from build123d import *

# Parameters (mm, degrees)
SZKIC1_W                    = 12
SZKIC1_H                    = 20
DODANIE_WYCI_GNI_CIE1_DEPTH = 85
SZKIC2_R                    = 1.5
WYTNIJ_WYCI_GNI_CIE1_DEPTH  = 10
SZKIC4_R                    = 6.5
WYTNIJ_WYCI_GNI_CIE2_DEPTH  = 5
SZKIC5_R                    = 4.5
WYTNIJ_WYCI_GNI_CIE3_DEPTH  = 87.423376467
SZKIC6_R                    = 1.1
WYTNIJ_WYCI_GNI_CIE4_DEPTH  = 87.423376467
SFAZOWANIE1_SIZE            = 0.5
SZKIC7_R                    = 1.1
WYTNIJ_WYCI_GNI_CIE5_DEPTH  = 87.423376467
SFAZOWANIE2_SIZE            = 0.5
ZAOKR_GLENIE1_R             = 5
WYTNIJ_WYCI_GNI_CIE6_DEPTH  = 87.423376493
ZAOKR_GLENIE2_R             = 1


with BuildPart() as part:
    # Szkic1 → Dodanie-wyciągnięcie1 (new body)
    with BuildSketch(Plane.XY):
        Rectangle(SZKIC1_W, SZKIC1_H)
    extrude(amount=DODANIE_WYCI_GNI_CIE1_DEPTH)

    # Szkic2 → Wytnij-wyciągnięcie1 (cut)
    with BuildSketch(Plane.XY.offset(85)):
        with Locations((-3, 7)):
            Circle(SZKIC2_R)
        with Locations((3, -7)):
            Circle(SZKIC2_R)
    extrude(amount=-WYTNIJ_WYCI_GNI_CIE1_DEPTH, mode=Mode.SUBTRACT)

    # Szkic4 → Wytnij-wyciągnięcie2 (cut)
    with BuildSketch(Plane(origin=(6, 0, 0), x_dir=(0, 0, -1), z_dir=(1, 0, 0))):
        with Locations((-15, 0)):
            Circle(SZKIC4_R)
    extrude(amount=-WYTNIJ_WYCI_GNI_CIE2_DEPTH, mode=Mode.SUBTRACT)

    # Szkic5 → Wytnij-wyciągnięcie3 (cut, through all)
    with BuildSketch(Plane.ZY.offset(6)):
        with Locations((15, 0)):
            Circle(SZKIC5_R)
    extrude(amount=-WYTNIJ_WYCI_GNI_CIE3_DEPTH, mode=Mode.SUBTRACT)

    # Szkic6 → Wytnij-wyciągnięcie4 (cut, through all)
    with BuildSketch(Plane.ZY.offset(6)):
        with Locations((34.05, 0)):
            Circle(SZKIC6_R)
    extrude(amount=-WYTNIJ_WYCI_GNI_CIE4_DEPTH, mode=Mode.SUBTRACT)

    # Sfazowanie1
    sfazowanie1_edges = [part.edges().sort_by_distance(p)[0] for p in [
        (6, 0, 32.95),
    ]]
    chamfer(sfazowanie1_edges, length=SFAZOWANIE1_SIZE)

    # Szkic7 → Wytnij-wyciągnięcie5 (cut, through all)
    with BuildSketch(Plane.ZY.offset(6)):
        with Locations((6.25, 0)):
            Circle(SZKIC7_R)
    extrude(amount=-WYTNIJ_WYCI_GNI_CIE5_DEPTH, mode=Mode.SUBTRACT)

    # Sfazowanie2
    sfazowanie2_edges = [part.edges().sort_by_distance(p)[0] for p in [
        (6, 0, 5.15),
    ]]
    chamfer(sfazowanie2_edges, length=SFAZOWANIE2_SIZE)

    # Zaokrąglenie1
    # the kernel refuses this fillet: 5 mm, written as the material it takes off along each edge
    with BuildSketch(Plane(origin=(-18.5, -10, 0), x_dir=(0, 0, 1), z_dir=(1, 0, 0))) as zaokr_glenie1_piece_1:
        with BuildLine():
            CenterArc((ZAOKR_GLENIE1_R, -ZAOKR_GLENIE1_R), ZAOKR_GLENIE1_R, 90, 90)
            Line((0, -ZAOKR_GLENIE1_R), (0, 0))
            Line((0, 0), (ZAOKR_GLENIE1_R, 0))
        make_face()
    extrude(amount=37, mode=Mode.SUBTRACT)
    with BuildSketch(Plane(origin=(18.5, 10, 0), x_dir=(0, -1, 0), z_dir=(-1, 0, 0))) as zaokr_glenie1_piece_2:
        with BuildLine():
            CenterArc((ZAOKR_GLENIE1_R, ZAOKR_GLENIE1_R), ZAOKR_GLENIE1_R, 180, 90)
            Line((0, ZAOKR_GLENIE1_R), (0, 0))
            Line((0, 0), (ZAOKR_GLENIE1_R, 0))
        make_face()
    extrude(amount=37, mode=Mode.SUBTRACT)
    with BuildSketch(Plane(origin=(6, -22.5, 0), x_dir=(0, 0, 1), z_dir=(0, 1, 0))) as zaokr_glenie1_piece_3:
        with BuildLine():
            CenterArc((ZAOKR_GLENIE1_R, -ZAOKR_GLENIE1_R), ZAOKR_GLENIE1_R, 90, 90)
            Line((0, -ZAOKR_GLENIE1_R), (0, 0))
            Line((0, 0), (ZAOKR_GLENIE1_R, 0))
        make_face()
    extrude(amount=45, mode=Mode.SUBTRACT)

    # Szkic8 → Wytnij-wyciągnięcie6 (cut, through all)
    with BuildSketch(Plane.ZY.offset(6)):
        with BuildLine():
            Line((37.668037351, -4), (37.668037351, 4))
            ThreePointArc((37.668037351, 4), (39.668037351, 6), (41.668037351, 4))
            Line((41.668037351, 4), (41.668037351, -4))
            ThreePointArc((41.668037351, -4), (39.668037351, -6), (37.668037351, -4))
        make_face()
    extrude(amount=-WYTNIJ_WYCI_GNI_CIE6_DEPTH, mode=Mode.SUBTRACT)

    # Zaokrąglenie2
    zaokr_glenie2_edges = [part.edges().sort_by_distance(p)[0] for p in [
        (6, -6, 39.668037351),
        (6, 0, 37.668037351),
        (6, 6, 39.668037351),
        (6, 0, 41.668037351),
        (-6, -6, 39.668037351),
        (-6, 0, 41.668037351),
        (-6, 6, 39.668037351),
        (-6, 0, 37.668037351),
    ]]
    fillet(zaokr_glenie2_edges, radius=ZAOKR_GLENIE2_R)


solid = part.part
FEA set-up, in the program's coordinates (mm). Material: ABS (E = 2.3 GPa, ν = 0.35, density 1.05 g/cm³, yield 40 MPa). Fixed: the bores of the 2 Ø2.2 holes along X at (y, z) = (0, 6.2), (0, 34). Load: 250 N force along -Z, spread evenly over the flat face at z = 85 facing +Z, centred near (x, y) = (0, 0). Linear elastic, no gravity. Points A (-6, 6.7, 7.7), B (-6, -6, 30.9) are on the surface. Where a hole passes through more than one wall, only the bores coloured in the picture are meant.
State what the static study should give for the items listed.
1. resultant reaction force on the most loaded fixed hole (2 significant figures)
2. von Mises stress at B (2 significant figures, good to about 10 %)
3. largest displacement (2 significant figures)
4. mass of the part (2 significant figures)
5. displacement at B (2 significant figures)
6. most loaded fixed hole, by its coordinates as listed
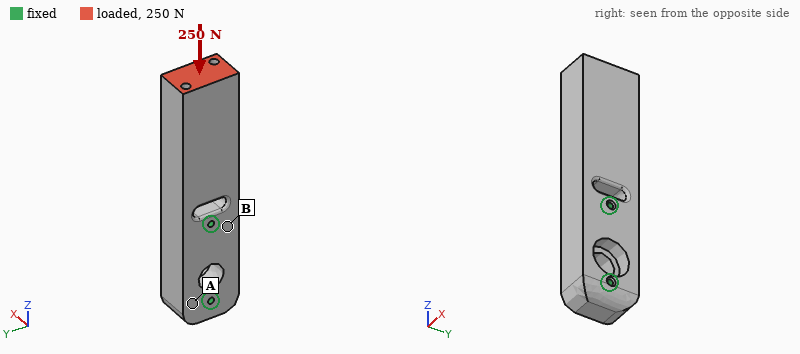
200 N
1.2 MPa
40 µm
19 g
6.7 µm
(0, 34)
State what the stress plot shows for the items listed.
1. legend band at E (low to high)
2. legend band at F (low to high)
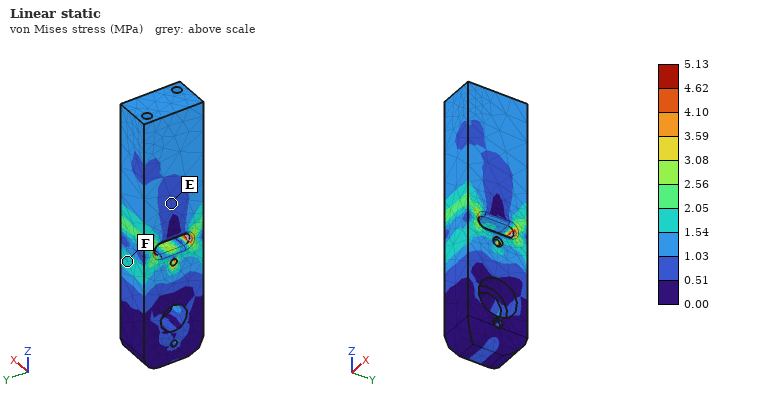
0.51 to 1.03 MPa
1.54 to 2.05 MPa
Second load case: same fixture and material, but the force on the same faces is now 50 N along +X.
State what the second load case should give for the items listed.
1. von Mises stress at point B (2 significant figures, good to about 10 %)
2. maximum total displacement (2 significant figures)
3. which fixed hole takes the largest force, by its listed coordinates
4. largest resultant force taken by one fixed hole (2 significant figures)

4.3 MPa
0.77 mm
(0, 34)
100 N
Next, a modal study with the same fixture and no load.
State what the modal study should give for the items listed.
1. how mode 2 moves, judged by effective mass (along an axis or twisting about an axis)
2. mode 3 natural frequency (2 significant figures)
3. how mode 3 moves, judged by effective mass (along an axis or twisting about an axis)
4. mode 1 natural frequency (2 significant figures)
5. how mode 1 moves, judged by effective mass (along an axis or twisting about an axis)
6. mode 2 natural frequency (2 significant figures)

along Y
3000 Hz
twisting about Z
680 Hz
along X
1100 Hz
